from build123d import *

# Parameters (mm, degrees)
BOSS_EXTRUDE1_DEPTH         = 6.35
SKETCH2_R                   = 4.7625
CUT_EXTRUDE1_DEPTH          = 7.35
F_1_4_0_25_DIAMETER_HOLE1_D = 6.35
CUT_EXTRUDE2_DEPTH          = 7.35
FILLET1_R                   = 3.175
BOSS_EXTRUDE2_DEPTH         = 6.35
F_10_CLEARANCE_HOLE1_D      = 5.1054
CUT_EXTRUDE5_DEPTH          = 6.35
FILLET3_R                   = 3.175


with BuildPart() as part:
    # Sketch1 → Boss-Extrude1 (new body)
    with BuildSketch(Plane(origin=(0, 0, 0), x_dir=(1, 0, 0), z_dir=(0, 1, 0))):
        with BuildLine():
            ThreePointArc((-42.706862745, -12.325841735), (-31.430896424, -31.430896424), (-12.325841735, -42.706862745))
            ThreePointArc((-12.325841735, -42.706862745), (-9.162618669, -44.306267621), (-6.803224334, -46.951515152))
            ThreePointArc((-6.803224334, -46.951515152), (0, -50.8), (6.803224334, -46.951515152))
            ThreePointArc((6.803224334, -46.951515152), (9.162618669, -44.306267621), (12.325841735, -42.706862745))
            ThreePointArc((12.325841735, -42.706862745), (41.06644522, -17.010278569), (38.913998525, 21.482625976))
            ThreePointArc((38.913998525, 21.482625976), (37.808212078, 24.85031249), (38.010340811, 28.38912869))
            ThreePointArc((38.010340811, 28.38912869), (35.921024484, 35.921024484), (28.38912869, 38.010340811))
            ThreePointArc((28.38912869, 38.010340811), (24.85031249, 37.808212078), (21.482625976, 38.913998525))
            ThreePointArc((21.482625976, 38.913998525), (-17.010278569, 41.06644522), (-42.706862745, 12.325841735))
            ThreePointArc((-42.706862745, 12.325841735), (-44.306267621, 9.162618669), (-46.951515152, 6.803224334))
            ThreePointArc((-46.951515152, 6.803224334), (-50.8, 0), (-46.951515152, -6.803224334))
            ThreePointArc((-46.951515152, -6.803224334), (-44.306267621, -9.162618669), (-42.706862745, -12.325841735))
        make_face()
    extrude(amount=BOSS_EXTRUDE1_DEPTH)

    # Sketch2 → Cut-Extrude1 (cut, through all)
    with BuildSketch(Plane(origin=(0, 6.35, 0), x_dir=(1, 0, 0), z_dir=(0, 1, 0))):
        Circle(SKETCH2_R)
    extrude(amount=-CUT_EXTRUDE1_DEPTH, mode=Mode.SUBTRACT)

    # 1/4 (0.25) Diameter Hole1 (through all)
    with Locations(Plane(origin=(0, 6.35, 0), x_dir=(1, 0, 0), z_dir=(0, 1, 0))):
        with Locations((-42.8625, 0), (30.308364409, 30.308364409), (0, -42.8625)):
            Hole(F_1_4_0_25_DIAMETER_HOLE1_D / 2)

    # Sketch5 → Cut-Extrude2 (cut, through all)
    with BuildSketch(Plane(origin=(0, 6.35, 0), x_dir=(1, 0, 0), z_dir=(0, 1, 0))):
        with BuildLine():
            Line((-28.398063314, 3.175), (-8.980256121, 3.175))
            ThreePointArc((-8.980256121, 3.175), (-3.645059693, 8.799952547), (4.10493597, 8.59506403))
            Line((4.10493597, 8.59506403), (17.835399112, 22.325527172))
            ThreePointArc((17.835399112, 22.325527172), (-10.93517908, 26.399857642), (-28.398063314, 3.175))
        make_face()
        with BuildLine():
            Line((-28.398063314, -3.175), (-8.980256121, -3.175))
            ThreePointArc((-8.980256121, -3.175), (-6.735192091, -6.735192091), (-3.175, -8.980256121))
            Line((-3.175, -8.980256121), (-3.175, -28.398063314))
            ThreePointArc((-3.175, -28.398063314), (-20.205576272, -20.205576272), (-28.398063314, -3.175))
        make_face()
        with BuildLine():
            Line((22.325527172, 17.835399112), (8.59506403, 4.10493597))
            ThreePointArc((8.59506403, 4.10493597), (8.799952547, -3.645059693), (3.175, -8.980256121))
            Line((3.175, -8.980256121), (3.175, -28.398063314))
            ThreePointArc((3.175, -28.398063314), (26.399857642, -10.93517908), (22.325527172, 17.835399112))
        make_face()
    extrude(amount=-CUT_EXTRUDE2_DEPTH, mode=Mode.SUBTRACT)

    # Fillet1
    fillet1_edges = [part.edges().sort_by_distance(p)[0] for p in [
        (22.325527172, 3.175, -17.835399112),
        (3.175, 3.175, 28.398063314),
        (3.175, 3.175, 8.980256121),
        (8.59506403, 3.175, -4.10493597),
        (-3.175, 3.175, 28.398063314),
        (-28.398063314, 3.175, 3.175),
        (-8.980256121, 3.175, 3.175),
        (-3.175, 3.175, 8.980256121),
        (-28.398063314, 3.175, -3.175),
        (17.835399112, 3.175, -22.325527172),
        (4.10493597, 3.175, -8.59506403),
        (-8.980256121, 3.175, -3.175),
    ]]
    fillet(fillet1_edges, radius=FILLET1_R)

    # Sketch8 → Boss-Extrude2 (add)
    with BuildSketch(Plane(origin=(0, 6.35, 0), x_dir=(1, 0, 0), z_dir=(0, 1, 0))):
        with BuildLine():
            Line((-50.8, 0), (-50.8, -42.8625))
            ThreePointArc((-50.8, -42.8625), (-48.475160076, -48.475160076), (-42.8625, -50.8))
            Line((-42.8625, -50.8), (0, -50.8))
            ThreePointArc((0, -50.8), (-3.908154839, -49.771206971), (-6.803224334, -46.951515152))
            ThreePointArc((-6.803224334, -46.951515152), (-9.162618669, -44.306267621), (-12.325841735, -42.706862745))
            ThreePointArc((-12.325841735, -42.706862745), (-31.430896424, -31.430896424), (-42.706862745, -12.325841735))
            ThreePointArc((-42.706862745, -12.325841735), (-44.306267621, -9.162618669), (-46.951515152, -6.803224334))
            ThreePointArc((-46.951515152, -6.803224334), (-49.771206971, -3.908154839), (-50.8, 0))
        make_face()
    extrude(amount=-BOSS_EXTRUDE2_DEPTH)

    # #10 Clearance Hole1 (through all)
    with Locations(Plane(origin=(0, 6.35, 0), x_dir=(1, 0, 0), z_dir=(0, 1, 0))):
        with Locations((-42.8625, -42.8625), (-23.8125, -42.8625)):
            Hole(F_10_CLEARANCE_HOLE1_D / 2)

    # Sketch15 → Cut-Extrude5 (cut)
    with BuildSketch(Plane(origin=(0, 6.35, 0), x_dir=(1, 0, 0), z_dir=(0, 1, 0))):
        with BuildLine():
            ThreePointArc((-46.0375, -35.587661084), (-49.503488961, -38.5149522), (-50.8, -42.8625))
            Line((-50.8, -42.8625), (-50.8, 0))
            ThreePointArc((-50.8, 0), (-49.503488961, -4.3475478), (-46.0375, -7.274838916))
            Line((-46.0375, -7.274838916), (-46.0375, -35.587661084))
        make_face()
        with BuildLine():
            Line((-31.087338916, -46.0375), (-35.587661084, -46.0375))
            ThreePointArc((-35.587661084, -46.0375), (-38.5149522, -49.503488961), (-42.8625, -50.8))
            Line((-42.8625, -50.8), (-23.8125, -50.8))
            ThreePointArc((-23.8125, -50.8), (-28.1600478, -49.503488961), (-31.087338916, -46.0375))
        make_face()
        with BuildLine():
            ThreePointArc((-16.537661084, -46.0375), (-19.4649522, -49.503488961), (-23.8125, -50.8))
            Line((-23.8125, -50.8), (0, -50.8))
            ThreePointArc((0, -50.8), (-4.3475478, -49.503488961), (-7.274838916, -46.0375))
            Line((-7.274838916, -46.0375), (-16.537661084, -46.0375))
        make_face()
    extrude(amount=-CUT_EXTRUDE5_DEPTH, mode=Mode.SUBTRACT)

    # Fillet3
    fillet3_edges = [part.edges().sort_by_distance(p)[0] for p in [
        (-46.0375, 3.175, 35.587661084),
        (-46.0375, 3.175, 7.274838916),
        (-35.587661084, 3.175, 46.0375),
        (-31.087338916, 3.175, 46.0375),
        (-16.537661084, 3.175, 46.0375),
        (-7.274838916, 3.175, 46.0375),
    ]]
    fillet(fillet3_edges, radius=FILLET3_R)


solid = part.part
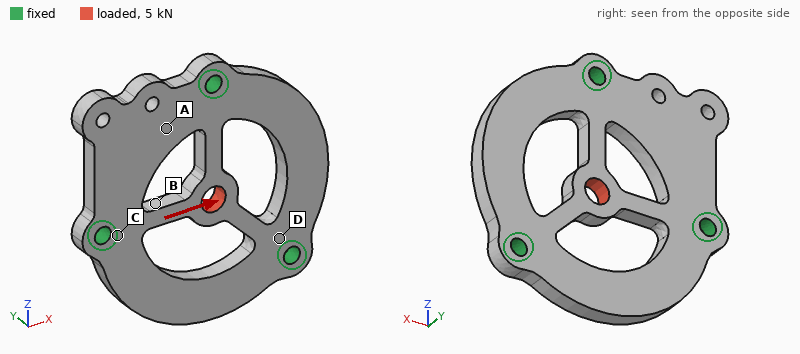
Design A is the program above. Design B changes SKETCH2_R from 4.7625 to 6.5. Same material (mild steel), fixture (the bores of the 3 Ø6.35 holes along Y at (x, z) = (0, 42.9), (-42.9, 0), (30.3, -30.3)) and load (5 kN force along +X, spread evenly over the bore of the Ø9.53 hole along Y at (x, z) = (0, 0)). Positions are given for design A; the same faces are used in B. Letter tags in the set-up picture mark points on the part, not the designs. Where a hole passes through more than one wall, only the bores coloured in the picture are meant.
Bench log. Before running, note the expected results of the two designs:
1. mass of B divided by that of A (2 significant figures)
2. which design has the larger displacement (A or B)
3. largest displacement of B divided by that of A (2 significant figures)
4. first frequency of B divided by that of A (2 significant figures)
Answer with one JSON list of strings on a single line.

["0.99", "B", "2.1", "1.00"]
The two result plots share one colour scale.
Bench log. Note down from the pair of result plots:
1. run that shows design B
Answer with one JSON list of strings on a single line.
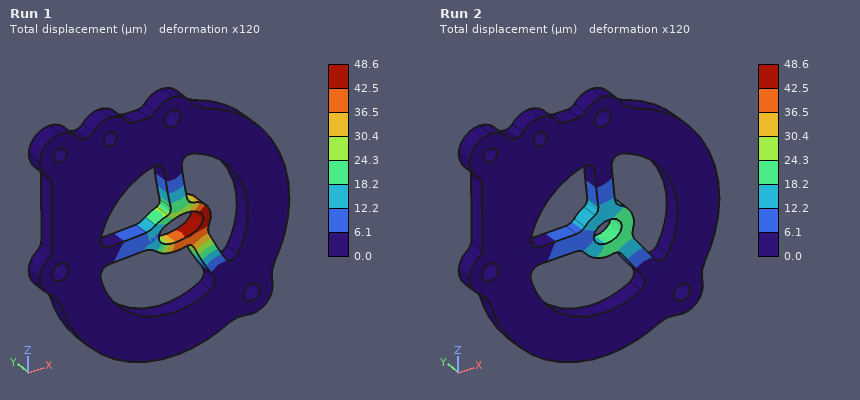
["Run 1"]
